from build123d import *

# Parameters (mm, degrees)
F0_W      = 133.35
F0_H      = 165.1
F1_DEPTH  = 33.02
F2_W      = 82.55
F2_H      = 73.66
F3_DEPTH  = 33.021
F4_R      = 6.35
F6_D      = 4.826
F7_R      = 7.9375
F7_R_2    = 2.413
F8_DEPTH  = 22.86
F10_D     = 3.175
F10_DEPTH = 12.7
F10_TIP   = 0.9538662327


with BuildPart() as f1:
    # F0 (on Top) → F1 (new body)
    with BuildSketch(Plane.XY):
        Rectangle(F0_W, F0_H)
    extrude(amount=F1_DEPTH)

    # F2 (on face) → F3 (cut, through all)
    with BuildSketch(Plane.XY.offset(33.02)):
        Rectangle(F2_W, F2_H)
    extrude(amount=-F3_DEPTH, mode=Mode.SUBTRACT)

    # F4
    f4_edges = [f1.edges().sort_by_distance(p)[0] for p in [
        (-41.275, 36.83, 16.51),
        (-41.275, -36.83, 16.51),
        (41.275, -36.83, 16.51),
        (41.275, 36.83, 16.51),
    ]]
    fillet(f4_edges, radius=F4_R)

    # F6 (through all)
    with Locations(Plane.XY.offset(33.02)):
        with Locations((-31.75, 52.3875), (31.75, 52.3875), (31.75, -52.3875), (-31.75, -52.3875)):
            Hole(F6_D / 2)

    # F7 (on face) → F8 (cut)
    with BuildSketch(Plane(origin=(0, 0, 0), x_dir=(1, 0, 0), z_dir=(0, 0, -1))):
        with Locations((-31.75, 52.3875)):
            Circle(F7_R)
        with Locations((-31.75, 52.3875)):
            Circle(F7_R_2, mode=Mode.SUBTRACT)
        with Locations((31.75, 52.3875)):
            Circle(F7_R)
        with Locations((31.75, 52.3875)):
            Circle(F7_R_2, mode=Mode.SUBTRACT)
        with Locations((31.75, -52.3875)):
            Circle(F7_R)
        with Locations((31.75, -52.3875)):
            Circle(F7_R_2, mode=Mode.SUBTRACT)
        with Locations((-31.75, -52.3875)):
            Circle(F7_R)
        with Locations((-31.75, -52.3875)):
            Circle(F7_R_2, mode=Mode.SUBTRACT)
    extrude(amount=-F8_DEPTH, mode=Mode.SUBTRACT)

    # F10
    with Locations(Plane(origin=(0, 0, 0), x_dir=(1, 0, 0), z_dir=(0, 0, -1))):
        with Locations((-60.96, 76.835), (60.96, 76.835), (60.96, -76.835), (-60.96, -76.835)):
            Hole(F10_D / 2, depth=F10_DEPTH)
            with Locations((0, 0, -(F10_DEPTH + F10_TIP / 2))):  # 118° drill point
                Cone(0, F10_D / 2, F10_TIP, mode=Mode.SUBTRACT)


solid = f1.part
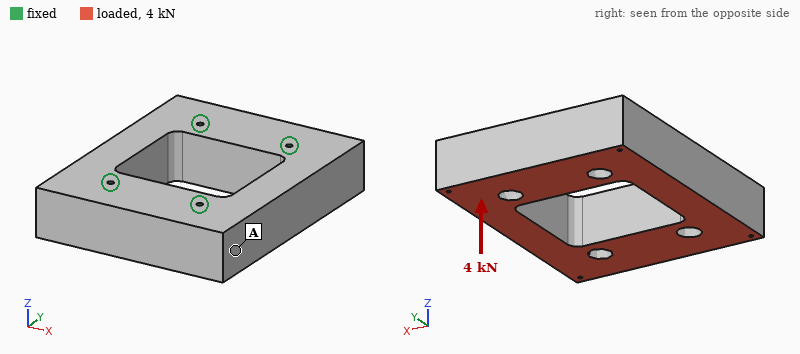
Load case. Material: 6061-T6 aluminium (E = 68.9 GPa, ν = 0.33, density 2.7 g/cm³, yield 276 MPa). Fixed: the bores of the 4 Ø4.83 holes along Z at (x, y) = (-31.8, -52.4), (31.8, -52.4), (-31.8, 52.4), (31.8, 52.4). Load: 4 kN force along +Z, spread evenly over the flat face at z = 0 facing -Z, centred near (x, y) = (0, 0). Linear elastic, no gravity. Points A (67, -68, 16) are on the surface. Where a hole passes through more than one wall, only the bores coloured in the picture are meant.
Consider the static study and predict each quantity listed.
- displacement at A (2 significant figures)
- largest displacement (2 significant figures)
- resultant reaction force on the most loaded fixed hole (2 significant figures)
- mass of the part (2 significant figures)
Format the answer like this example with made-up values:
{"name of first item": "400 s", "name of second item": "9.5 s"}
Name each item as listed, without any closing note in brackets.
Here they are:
{"displacement at A": "2.7 µm", "largest displacement": "3.8 µm", "resultant reaction force on the most loaded fixed hole": "1.0 kN", "mass of the part": "1.4 kg"}
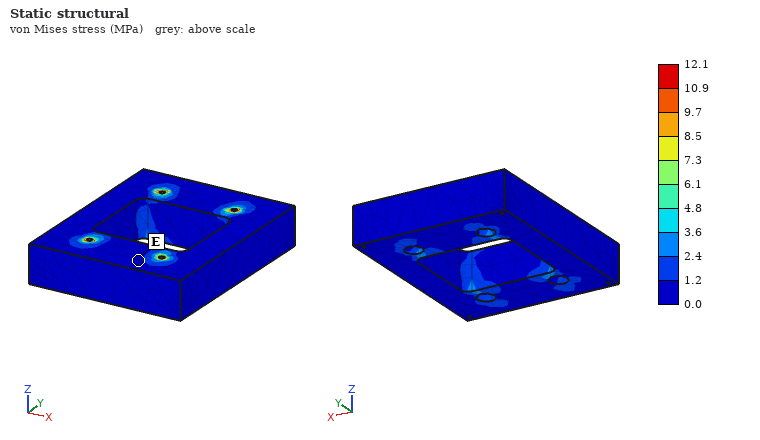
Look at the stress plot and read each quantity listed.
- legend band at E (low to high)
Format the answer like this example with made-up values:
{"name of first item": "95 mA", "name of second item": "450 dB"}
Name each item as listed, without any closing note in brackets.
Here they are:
{"legend band at E": "0.0 to 1.2 MPa"}
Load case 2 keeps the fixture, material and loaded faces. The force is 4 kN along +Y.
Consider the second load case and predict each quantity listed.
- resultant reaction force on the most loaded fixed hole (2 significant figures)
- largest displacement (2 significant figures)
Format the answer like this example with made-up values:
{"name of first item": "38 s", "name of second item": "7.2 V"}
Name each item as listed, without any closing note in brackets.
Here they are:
{"resultant reaction force on the most loaded fixed hole": "1.1 kN", "largest displacement": "6.6 µm"}
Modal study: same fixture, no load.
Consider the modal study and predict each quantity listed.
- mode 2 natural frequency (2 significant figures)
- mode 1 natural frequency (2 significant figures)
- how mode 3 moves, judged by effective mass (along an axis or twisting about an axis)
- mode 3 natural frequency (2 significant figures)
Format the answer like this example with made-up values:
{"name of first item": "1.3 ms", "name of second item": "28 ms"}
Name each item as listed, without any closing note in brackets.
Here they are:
{"mode 2 natural frequency": "4700 Hz", "mode 1 natural frequency": "4300 Hz", "how mode 3 moves, judged by effective mass": "along Y", "mode 3 natural frequency": "4900 Hz"}
